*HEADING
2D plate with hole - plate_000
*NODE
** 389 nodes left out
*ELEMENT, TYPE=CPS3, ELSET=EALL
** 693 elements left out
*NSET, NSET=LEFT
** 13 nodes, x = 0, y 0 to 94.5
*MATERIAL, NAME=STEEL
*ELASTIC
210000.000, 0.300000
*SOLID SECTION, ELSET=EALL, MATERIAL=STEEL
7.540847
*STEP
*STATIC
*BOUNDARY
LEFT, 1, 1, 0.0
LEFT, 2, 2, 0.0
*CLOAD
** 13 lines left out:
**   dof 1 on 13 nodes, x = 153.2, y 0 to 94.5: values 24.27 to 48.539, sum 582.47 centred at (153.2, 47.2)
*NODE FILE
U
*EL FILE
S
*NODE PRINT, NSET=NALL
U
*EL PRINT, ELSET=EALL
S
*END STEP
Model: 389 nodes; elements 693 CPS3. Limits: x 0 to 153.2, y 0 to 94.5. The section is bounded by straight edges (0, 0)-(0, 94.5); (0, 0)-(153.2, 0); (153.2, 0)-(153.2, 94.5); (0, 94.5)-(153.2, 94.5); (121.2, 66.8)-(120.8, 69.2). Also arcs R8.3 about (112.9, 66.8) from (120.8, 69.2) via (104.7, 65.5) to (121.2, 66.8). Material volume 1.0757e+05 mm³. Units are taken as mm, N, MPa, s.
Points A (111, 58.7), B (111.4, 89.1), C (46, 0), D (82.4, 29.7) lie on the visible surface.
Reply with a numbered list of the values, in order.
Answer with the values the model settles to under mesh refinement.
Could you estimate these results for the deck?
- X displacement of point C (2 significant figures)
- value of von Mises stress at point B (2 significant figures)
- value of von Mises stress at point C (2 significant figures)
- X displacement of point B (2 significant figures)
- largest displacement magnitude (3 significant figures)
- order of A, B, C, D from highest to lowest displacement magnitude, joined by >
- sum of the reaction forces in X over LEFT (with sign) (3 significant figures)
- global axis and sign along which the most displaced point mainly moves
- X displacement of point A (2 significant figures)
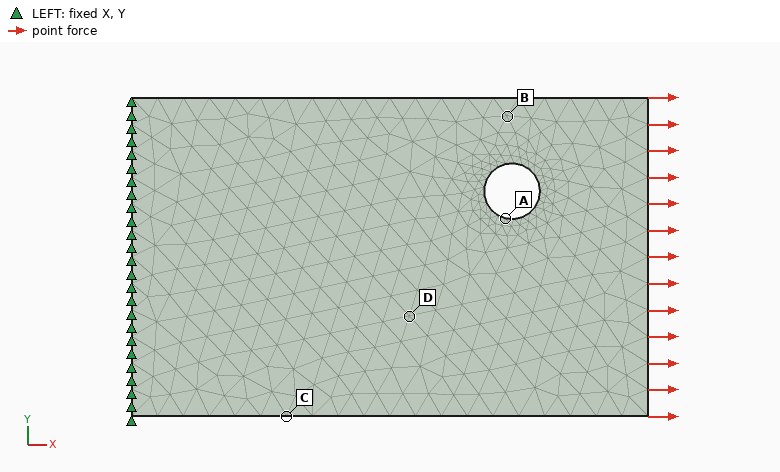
1. 1.8e-04 mm
2. 0.88 MPa
3. 0.78 MPa
4. 4.6e-04 mm
5. 6.95e-04 mm
6. B > A > D > C
7. -582 N
8. +X
9. 4.3e-04 mm
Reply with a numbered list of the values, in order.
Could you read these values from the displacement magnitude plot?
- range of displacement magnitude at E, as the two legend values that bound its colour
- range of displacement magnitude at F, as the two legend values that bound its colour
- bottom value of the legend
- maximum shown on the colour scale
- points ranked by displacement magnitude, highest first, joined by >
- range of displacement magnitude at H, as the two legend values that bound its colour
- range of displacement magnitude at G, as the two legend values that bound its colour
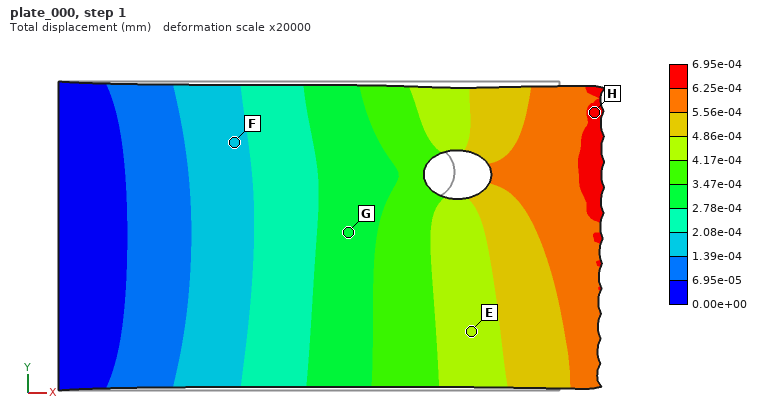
1. 4.17e-04 to 4.86e-04 mm
2. 1.39e-04 to 2.08e-04 mm
3. 0.00e+00 mm
4. 6.95e-04 mm
5. H > E > G > F
6. 6.25e-04 to 6.95e-04 mm
7. 2.78e-04 to 3.47e-04 mm
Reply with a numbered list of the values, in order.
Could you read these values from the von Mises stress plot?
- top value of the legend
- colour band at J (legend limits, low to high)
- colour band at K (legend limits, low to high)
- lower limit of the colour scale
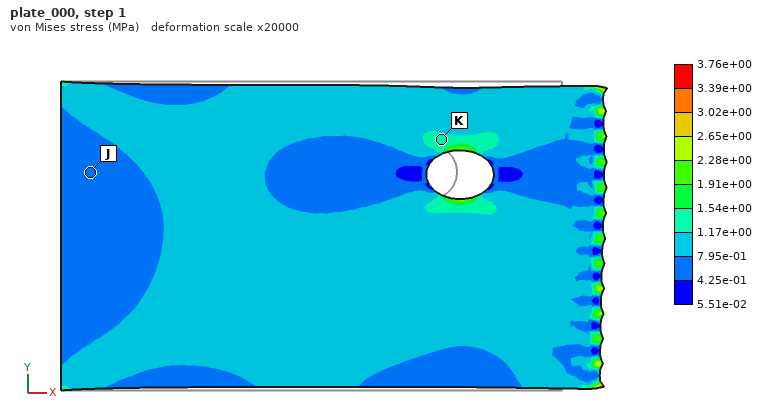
1. 3.76e+00 MPa
2. 4.25e-01 to 7.95e-01 MPa
3. 1.17e+00 to 1.54e+00 MPa
4. 5.51e-02 MPa
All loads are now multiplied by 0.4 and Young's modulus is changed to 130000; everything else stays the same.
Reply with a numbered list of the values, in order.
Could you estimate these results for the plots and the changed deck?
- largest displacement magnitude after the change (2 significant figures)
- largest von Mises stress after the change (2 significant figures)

1. 4.5e-04 mm
2. 1.5 MPa
